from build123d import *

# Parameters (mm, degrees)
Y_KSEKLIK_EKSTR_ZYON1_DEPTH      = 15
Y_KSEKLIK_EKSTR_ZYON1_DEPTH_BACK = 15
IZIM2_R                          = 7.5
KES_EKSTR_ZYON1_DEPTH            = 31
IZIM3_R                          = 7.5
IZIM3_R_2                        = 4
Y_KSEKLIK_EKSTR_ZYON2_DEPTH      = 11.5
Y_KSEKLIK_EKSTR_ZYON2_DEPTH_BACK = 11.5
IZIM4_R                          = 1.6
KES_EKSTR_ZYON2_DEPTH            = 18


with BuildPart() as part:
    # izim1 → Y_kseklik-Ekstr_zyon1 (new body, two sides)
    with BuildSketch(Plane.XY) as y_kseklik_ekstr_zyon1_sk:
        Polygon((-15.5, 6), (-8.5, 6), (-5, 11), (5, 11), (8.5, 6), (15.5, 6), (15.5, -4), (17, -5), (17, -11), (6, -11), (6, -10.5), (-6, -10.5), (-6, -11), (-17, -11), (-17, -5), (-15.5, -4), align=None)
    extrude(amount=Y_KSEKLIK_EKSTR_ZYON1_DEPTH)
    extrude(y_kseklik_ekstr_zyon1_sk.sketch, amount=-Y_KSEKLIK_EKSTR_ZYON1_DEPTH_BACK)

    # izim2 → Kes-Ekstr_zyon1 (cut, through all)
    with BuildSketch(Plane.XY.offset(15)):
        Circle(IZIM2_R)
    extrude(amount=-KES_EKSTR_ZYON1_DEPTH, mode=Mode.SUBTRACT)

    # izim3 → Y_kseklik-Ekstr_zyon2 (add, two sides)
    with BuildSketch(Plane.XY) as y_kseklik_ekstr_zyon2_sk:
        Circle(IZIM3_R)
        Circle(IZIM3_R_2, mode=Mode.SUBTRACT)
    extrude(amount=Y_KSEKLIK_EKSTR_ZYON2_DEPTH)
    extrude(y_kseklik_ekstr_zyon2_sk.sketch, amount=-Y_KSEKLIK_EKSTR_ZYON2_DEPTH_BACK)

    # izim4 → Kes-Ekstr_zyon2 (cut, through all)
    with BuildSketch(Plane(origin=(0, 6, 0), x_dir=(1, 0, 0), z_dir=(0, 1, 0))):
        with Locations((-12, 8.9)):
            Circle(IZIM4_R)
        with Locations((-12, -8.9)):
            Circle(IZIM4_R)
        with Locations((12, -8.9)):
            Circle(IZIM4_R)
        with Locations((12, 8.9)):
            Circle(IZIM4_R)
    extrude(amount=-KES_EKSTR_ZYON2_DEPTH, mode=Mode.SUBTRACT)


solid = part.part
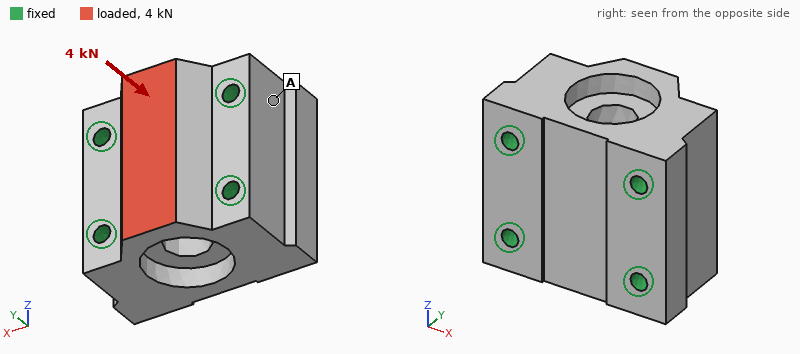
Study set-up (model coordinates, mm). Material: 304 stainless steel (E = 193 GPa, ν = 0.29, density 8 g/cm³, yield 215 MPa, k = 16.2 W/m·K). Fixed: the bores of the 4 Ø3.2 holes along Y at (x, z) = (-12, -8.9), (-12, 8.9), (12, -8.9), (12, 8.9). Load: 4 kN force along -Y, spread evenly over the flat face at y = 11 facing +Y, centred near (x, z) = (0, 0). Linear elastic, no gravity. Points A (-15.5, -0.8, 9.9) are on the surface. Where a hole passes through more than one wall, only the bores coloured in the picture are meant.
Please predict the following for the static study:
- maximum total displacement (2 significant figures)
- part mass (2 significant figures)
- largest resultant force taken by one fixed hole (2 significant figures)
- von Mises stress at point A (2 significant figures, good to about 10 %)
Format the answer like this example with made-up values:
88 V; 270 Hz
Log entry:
2.4 µm; 120 g; 1.1 kN; 3.1 MPa
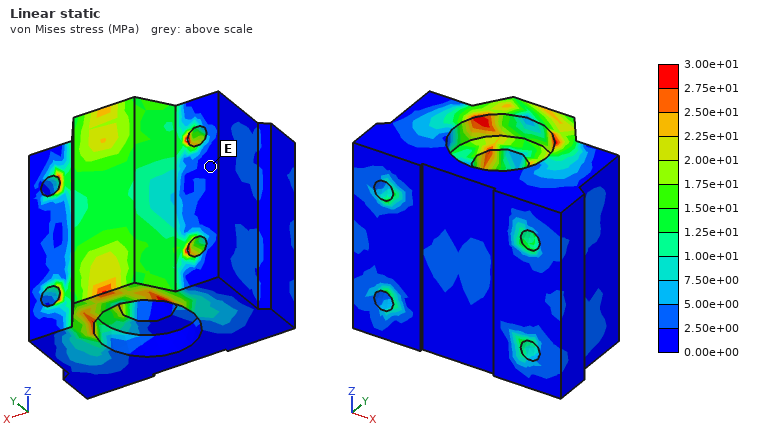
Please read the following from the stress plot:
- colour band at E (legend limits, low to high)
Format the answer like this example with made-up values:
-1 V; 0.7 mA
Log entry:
0.00e+00 to 2.50e+00 MPa
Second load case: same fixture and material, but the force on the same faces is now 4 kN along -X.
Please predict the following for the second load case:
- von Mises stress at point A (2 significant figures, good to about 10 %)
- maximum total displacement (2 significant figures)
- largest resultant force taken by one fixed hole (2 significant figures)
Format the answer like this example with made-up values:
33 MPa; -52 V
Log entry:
5.0 MPa; 1.8 µm; 1.3 kN
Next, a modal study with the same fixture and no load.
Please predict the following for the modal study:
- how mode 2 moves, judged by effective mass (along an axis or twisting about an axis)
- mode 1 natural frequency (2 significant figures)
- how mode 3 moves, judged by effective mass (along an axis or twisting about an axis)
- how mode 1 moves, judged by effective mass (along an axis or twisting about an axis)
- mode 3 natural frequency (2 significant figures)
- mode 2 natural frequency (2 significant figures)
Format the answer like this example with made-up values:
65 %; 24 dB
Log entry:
along Y; 46 kHz; along Z; along Z; 61 kHz; 52 kHz
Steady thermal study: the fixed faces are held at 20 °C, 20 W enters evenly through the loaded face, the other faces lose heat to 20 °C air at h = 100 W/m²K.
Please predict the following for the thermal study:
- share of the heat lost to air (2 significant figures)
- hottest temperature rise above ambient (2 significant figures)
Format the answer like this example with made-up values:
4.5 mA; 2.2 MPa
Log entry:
16 %; 44 K
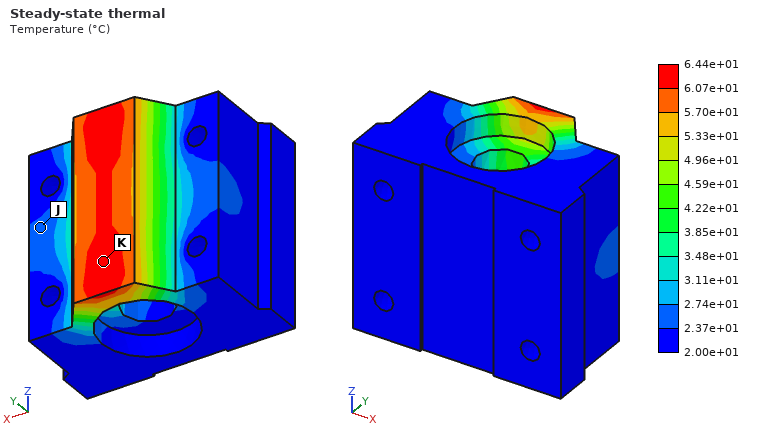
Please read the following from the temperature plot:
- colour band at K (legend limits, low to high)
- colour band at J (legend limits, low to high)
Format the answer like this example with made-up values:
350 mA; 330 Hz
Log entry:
6.07e+01 to 6.44e+01 °C; 2.37e+01 to 2.74e+01 °C
